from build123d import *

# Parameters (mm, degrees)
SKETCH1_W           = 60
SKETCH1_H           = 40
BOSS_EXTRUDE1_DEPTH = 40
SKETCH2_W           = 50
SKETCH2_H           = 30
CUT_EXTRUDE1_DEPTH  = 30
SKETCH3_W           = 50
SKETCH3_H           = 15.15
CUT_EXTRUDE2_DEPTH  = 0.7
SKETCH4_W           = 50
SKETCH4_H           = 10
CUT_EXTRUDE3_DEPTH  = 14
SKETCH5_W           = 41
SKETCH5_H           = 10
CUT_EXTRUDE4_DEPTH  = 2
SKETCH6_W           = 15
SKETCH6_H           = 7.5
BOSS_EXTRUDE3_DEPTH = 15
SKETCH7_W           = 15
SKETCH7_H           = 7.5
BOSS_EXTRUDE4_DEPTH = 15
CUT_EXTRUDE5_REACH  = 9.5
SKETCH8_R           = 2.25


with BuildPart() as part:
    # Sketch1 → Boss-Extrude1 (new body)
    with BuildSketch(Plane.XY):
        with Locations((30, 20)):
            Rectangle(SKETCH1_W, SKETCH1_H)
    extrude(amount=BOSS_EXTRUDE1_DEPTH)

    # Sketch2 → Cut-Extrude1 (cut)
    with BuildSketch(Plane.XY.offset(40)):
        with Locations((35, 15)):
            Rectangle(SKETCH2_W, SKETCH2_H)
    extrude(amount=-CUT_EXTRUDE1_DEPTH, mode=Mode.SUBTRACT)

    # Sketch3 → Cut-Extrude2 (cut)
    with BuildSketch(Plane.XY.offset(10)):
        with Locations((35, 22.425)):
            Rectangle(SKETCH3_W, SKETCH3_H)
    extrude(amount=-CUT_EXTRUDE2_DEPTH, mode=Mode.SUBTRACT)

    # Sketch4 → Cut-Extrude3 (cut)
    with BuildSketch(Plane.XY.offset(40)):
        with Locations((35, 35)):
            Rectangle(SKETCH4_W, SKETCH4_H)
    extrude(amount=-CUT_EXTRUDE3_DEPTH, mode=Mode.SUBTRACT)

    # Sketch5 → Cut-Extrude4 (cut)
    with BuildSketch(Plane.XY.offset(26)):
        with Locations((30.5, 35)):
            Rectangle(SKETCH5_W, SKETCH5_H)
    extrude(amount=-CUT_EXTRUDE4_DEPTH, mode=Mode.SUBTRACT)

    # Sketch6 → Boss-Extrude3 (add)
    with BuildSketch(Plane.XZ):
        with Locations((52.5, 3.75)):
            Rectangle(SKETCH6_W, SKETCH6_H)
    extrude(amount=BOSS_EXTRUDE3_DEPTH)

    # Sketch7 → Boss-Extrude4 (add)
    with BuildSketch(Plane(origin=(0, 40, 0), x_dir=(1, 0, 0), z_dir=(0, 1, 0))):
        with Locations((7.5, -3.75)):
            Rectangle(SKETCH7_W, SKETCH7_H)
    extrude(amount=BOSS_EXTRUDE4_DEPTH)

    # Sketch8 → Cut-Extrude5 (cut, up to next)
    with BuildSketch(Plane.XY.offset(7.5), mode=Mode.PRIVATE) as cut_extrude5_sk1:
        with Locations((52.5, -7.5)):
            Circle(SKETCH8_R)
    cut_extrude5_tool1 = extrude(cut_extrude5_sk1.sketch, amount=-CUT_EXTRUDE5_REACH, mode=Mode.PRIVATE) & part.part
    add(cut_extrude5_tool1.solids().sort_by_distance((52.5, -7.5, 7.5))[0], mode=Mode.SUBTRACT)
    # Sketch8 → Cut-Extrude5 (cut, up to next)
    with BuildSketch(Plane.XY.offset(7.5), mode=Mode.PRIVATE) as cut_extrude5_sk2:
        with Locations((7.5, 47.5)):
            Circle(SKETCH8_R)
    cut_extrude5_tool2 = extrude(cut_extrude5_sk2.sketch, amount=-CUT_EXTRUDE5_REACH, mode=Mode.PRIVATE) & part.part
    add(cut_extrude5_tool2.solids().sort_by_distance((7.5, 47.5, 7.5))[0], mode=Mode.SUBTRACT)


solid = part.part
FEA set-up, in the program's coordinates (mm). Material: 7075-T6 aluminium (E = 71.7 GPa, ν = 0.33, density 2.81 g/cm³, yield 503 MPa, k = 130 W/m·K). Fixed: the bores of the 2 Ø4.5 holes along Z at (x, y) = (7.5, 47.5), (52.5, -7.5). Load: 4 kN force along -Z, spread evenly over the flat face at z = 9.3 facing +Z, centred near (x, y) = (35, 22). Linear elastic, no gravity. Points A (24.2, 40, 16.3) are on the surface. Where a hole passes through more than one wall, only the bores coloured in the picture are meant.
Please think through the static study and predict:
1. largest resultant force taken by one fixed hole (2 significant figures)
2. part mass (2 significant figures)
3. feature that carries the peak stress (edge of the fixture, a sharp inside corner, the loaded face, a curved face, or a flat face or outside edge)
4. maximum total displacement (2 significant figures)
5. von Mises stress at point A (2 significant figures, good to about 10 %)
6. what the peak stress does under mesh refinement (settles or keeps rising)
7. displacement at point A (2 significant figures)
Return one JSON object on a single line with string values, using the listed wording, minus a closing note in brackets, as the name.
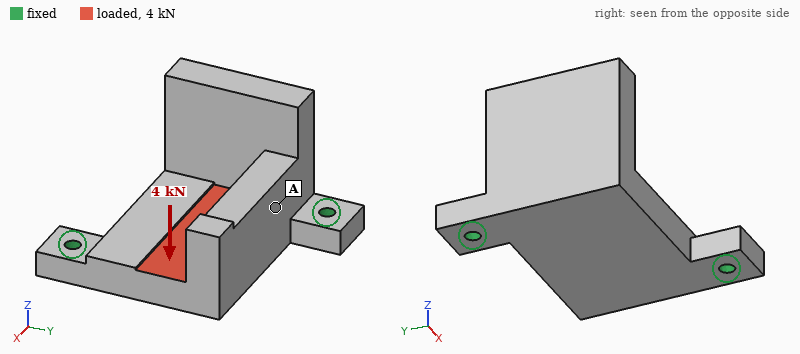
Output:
{"largest resultant force taken by one fixed hole": "2.2 kN", "part mass": "130 g", "feature that carries the peak stress": "edge of the fixture", "maximum total displacement": "0.19 mm", "von Mises stress at point A": "24 MPa", "what the peak stress does under mesh refinement": "keeps rising", "displacement at point A": "0.071 mm"}
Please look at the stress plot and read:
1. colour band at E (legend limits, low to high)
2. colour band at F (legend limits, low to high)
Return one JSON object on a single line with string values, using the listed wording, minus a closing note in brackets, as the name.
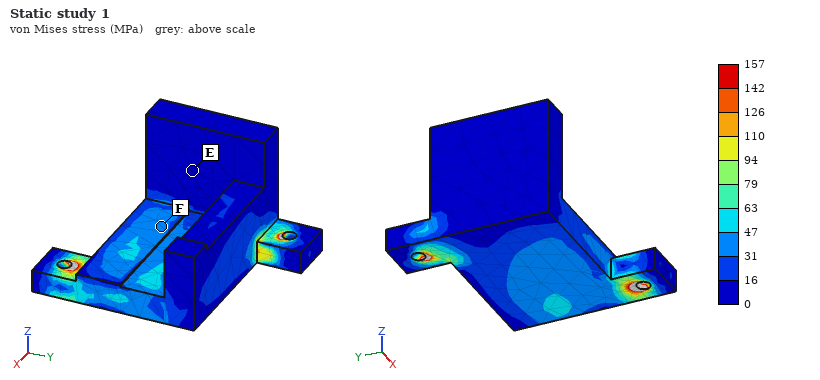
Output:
{"colour band at E": "0 to 16 MPa", "colour band at F": "31 to 47 MPa"}
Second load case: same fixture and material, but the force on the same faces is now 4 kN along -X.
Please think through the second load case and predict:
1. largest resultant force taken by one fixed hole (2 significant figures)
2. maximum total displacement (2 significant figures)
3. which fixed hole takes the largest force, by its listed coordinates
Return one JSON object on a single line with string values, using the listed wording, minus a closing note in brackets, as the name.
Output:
{"largest resultant force taken by one fixed hole": "2.1 kN", "maximum total displacement": "0.12 mm", "which fixed hole takes the largest force, by its listed coordinates": "(7.5, 47.5)"}
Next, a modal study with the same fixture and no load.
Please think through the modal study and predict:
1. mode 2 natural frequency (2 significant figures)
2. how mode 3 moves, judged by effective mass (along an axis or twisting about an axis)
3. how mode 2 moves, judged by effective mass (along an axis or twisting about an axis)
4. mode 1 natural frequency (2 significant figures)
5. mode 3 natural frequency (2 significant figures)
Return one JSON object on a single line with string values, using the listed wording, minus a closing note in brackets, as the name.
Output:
{"mode 2 natural frequency": "3600 Hz", "how mode 3 moves, judged by effective mass": "along X", "how mode 2 moves, judged by effective mass": "along Z", "mode 1 natural frequency": "1800 Hz", "mode 3 natural frequency": "6100 Hz"}
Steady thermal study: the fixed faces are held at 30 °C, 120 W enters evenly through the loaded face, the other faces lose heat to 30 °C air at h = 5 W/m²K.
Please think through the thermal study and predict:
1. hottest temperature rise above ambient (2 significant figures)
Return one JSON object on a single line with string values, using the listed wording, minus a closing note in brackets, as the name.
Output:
{"hottest temperature rise above ambient": "73 K"}
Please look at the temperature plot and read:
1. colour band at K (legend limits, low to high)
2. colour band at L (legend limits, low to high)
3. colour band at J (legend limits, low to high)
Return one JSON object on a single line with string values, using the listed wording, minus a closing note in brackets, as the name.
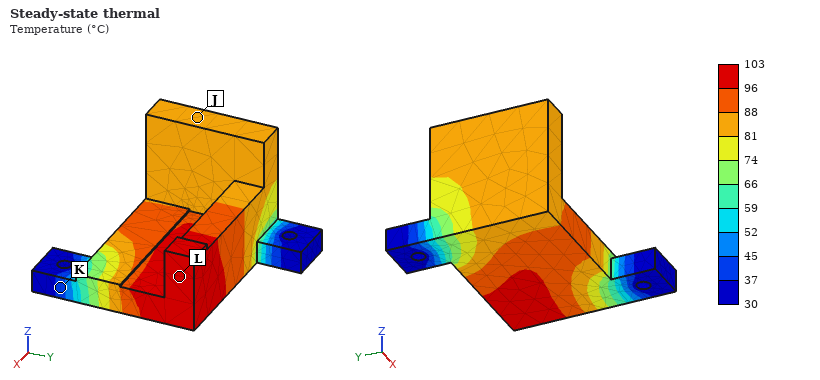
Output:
{"colour band at K": "37 to 45 °C", "colour band at L": "96 to 103 °C", "colour band at J": "81 to 88 °C"}
